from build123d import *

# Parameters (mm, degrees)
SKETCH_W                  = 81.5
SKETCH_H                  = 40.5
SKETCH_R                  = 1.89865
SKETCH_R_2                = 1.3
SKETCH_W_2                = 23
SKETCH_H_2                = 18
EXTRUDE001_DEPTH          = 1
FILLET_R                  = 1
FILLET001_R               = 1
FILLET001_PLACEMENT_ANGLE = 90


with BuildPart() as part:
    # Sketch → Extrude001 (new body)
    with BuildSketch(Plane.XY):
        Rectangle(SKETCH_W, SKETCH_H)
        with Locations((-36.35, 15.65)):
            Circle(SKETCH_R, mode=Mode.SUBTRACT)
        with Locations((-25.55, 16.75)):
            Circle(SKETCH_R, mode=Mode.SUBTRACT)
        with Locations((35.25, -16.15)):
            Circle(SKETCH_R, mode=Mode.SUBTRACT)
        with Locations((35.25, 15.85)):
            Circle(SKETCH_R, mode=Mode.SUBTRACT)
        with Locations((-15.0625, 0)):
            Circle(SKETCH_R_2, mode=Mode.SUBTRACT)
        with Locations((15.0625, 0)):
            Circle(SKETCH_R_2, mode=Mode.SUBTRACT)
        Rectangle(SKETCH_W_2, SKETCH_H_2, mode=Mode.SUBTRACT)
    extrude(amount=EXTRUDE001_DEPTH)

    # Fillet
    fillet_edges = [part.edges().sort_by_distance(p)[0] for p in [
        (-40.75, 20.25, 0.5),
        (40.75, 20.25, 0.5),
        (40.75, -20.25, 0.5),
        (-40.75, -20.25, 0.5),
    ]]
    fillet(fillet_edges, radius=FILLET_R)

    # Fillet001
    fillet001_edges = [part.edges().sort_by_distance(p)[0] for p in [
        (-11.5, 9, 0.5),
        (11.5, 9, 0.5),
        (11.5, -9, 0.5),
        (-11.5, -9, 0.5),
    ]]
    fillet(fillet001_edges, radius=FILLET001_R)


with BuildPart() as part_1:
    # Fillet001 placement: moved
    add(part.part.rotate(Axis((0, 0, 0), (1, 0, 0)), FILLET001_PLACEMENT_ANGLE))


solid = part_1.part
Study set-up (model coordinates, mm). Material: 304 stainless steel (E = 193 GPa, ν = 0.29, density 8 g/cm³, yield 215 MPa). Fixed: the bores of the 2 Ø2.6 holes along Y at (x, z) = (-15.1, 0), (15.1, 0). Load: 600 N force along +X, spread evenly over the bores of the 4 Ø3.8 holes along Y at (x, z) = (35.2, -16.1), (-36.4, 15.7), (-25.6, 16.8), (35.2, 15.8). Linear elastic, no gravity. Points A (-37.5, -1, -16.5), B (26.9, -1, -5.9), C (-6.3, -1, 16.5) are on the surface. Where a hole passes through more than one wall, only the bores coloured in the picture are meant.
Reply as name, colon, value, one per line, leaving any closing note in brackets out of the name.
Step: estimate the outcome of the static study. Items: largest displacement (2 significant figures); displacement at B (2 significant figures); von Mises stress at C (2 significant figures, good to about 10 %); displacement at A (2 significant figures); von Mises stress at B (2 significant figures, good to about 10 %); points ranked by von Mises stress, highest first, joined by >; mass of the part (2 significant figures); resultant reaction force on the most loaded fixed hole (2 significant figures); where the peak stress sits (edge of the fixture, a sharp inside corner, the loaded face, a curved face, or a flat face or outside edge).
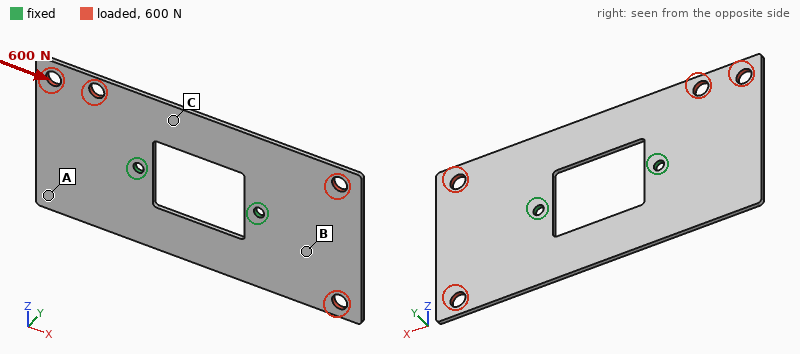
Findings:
largest displacement: 17 µm
displacement at B: 3.8 µm
von Mises stress at C: 22 MPa
displacement at A: 11 µm
von Mises stress at B: 12 MPa
points ranked by von Mises stress, highest first, joined by >: C > B > A
mass of the part: 23 g
resultant reaction force on the most loaded fixed hole: 320 N
where the peak stress sits: edge of the fixture
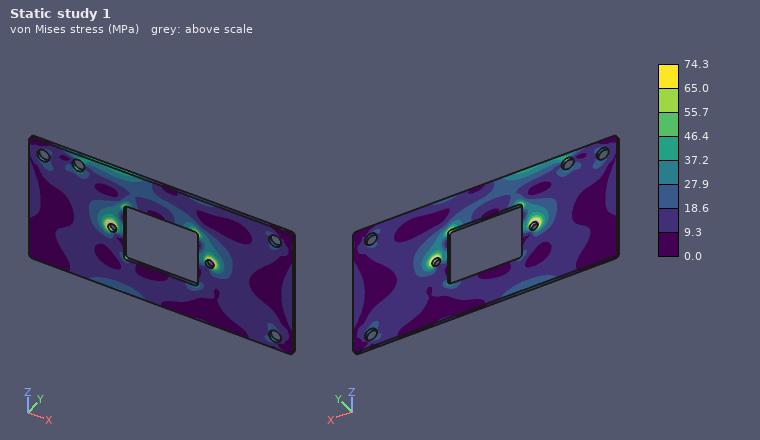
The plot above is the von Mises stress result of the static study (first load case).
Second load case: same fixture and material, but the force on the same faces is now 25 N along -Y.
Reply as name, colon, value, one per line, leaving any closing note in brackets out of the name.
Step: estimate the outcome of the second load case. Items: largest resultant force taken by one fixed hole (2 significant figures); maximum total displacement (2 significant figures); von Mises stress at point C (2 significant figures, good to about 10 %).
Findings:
largest resultant force taken by one fixed hole: 13 N
maximum total displacement: 0.18 mm
von Mises stress at point C: 20 MPa
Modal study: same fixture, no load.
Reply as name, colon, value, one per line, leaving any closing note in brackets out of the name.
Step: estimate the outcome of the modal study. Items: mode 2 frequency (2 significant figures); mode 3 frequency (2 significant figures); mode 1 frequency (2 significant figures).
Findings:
mode 2 frequency: 1000 Hz
mode 3 frequency: 1000 Hz
mode 1 frequency: 990 Hz
